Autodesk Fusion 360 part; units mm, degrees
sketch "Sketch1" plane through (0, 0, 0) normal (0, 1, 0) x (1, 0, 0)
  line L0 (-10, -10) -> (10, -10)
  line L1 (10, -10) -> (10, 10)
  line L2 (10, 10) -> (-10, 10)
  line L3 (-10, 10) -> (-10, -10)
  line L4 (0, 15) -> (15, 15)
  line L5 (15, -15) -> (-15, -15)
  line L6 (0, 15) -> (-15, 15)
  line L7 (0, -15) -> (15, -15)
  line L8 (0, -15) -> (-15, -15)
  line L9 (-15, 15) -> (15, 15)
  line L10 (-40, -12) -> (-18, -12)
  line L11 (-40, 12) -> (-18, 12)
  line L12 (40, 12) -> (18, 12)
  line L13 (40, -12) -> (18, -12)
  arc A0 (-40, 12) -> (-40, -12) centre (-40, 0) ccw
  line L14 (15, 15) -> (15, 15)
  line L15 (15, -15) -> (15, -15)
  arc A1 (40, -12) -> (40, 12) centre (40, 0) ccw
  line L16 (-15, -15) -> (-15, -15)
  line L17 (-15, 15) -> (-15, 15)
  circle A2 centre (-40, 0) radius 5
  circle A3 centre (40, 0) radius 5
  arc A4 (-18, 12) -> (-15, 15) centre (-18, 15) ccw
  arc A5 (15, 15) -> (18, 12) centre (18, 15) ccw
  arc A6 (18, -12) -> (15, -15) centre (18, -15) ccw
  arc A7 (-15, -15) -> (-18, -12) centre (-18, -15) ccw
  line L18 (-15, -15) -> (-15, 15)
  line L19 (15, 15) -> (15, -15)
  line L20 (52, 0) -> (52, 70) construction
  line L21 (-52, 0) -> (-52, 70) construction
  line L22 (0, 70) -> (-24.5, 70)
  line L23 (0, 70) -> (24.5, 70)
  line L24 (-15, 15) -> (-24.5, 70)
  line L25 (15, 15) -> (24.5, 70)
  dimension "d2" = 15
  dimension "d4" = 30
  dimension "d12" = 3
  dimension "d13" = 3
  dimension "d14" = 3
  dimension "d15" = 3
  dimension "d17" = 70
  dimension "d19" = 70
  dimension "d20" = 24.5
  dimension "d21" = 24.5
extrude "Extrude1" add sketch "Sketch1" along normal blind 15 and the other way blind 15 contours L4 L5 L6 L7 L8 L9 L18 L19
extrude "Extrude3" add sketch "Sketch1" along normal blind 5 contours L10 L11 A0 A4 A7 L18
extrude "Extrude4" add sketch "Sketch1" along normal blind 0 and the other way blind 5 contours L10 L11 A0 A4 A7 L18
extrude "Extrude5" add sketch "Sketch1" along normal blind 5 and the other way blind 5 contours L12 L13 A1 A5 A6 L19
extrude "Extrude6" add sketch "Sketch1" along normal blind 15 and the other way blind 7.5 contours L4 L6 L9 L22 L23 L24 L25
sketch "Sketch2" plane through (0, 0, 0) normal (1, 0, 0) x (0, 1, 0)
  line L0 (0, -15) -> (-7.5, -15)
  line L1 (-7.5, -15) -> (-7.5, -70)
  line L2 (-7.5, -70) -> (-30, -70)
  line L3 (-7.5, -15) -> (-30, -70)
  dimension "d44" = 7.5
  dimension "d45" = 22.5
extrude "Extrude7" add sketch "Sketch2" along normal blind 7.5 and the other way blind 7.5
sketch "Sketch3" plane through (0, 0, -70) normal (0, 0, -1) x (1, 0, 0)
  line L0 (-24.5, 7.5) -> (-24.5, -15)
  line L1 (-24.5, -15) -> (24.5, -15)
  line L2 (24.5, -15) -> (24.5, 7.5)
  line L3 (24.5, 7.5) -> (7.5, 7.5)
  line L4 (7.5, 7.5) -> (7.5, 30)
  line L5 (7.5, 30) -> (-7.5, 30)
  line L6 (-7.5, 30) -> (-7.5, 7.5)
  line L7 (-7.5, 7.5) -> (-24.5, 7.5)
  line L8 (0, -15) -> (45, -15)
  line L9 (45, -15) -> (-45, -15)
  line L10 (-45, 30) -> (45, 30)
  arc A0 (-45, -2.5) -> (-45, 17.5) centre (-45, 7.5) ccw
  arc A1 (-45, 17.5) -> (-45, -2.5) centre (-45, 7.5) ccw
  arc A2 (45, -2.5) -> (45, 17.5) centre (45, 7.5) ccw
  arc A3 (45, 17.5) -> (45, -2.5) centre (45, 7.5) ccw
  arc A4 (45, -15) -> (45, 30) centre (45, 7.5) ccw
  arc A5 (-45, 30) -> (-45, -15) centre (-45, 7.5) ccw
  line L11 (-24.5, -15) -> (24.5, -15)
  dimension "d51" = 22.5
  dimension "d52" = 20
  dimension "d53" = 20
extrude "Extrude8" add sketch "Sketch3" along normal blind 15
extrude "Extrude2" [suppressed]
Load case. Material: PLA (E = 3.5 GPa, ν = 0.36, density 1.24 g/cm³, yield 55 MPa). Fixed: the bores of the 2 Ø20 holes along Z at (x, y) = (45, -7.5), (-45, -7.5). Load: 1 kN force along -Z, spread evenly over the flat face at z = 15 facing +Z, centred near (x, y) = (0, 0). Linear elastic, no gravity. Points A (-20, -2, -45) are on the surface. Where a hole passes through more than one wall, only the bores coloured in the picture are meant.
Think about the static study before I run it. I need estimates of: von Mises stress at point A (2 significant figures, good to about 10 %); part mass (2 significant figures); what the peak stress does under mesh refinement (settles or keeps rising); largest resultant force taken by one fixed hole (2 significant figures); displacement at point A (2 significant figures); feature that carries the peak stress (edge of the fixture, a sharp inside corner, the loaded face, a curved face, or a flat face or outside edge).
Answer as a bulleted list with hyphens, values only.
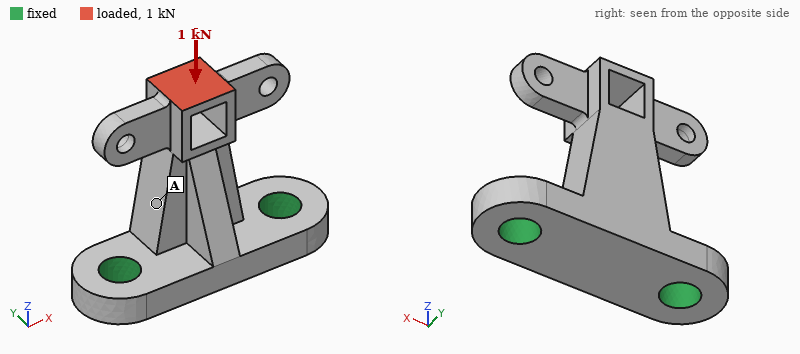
- 1.2 MPa
- 200 g
- keeps rising
- 530 N
- 0.047 mm
- a sharp inside corner
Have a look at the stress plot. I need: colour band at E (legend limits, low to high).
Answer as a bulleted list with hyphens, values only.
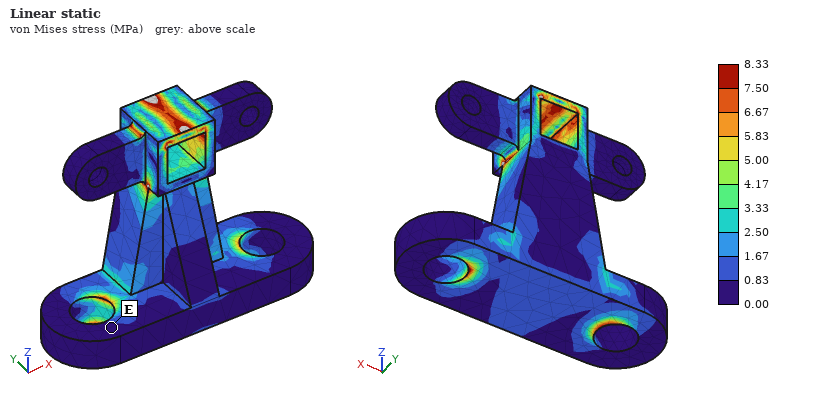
- 0.00 to 0.83 MPa
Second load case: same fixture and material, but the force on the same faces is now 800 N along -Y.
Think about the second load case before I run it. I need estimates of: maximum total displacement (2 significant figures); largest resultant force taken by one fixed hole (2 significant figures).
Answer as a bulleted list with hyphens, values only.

- 2.1 mm
- 410 N
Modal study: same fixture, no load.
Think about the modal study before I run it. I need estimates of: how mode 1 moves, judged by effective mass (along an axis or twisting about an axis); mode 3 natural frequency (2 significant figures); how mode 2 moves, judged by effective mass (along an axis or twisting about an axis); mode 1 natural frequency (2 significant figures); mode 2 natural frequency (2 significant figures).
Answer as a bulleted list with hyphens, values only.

- along Y
- 1100 Hz
- along X
- 560 Hz
- 790 Hz
